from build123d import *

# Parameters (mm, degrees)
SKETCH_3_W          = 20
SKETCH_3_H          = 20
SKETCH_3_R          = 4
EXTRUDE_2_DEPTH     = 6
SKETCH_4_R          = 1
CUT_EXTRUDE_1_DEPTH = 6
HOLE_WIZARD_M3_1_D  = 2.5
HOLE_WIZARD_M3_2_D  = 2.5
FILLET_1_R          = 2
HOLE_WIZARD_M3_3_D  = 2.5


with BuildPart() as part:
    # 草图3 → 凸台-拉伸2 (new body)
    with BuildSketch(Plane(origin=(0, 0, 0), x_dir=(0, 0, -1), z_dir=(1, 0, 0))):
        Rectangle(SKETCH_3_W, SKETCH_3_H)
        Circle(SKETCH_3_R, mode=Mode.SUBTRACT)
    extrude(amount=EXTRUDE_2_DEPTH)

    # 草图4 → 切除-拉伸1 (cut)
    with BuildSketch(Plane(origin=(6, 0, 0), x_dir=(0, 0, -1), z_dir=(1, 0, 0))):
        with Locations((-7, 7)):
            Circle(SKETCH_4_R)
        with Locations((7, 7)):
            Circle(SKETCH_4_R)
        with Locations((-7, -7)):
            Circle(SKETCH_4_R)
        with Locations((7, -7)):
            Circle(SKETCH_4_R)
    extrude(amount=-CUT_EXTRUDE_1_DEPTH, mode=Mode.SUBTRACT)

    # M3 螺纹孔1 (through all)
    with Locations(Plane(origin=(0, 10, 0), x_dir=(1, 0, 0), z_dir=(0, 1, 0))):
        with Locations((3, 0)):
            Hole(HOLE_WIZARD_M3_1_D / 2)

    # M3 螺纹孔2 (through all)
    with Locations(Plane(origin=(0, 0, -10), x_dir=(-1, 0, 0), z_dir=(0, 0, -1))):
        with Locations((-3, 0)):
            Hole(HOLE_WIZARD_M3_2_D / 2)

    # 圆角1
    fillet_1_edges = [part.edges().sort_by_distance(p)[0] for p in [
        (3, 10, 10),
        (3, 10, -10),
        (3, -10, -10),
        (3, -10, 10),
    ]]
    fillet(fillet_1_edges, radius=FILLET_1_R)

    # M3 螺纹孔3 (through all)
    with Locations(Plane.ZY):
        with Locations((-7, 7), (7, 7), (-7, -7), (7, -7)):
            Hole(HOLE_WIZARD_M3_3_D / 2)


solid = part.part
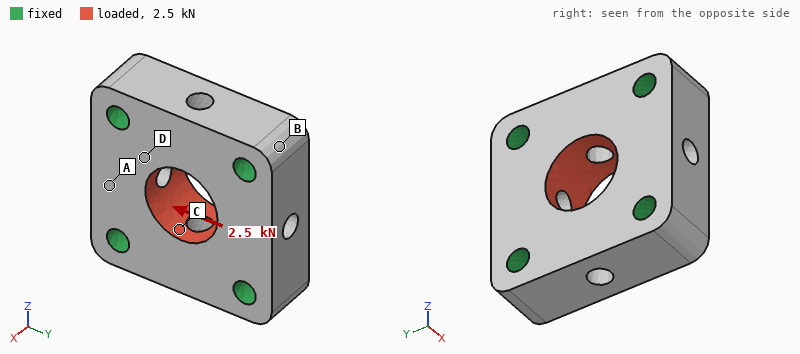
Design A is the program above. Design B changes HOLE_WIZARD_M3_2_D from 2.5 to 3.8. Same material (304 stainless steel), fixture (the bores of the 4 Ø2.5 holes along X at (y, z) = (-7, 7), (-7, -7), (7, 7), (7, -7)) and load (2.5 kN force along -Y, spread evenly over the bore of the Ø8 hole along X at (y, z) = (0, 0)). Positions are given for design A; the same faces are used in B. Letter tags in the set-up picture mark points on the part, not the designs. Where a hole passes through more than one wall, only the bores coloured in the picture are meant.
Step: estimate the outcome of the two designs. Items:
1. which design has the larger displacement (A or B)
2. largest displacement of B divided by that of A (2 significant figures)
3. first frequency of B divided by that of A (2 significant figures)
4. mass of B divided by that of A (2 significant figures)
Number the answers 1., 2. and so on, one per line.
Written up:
1. B
2. 1.2
3. 1.00
4. 0.96
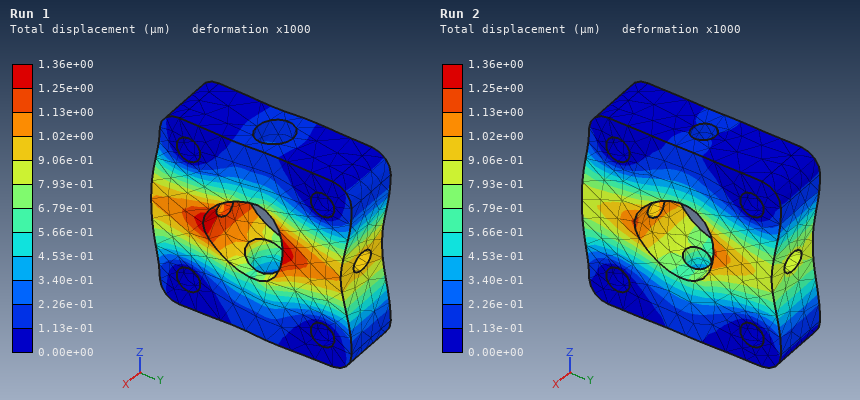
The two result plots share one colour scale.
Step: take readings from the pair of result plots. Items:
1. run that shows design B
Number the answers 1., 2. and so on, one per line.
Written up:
1. Run 1
